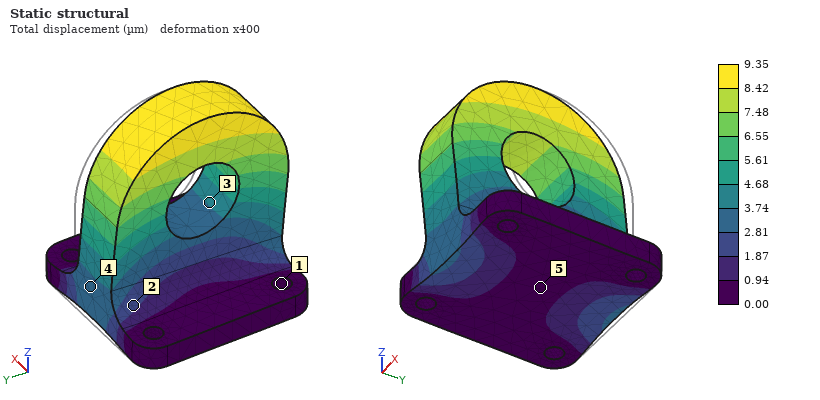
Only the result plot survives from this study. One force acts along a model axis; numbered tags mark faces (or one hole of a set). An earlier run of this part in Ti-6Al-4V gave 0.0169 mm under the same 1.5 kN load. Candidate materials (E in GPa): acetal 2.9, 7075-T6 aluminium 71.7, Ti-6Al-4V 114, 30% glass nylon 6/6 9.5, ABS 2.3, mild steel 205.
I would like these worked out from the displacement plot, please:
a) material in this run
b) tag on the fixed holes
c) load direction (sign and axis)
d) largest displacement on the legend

mild steel
1
-Y
9.35 µm
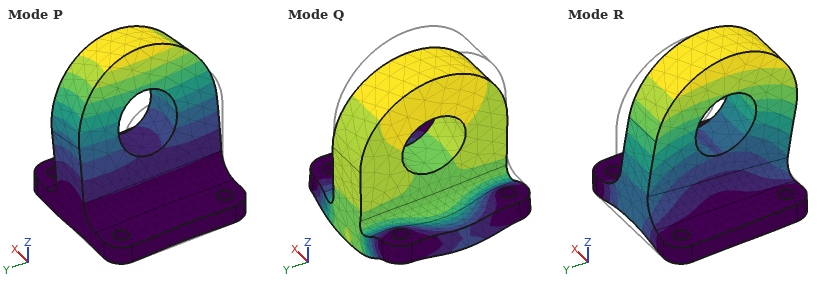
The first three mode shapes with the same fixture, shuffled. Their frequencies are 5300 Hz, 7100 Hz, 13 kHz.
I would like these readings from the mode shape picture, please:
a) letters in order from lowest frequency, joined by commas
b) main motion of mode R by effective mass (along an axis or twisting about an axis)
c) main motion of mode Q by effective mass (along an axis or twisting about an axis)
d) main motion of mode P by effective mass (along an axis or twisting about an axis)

P, R, Q
along Y
along Z
along X
